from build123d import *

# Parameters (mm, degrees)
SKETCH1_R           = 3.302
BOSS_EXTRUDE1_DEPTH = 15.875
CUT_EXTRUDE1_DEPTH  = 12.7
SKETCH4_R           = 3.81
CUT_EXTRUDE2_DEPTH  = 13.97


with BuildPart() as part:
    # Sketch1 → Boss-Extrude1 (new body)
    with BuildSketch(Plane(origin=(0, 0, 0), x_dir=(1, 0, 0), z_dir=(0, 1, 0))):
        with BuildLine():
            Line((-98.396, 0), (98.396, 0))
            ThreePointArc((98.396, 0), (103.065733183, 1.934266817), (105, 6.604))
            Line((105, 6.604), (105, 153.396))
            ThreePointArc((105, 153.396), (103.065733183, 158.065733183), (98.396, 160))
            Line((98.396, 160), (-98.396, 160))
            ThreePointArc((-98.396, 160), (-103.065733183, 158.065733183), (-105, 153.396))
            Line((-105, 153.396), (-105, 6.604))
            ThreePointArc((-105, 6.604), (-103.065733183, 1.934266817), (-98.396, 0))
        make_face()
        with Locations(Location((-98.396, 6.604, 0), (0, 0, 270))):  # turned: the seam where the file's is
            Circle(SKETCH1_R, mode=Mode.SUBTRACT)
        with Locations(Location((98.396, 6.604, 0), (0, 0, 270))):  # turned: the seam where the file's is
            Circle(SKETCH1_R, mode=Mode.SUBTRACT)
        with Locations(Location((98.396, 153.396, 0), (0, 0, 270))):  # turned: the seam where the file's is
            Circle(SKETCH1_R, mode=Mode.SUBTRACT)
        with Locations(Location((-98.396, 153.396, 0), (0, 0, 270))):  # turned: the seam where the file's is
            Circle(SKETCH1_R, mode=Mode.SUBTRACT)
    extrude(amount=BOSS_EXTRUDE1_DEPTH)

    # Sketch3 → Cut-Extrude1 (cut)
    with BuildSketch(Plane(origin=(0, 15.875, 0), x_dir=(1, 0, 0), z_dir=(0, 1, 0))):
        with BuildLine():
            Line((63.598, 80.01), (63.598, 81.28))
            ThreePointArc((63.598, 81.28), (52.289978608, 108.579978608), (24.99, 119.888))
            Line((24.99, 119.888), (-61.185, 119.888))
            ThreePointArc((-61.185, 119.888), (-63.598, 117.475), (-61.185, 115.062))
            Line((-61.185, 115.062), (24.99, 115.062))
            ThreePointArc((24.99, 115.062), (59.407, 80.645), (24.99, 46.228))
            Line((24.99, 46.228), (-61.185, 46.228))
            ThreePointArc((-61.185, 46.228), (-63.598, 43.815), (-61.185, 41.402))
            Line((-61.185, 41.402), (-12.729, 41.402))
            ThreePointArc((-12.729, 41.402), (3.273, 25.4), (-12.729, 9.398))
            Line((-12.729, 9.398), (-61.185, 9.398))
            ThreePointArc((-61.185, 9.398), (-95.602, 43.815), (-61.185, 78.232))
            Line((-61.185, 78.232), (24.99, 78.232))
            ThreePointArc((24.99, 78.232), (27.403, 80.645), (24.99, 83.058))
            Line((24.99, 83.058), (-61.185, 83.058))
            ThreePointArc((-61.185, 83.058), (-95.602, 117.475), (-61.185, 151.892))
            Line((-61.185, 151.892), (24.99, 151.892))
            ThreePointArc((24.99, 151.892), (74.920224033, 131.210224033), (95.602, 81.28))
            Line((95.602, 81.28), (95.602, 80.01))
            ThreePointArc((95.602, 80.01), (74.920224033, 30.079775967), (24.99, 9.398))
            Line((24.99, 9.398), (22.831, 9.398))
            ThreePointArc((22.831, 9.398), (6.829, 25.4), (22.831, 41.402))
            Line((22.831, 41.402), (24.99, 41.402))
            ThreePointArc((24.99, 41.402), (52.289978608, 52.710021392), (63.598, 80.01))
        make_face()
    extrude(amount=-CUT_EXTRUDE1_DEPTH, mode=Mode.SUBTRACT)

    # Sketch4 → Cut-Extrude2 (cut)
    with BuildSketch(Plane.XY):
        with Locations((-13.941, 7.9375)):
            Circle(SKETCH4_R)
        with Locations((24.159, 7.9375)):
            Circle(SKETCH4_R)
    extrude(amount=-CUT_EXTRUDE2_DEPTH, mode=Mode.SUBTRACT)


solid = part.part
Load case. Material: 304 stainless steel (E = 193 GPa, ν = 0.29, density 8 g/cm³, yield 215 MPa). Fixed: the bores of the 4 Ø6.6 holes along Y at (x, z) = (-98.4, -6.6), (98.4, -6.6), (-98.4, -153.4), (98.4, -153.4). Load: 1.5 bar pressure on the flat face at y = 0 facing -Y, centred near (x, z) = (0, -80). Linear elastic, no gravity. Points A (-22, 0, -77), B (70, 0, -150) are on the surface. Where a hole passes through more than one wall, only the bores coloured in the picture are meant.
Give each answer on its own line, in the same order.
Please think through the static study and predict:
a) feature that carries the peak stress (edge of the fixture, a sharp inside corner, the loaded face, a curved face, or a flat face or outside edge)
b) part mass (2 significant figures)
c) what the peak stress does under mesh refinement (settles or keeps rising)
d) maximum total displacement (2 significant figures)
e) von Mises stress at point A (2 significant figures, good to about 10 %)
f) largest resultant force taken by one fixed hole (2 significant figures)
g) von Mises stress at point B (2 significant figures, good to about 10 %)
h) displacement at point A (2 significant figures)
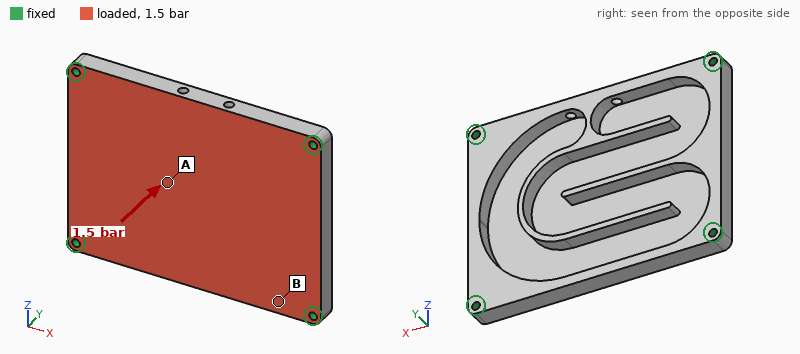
edge of the fixture
2.0 kg
keeps rising
0.11 mm
17 MPa
1.6 kN
8.6 MPa
0.097 mm
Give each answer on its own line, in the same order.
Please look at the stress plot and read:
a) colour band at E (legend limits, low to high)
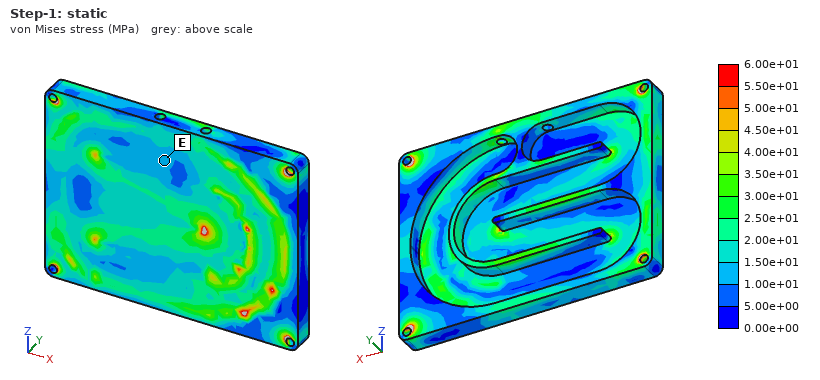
1.00e+01 to 1.50e+01 MPa
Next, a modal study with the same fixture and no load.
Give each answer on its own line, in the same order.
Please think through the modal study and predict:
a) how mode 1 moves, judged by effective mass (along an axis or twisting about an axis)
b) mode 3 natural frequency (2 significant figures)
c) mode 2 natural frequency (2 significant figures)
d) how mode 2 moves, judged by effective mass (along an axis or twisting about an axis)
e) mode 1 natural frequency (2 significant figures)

along Y
2200 Hz
1800 Hz
twisting about X
1200 Hz
